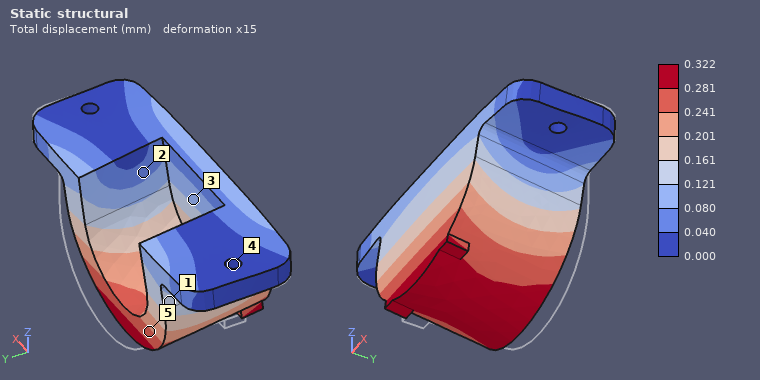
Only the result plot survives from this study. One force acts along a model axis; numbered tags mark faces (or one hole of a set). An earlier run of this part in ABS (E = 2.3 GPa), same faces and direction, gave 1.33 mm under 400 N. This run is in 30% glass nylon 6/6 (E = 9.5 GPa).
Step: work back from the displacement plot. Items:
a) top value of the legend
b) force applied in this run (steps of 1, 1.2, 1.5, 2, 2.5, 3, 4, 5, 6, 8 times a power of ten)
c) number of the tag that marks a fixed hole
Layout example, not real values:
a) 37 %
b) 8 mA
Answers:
a) 0.322 mm
b) 400 N
c) 4
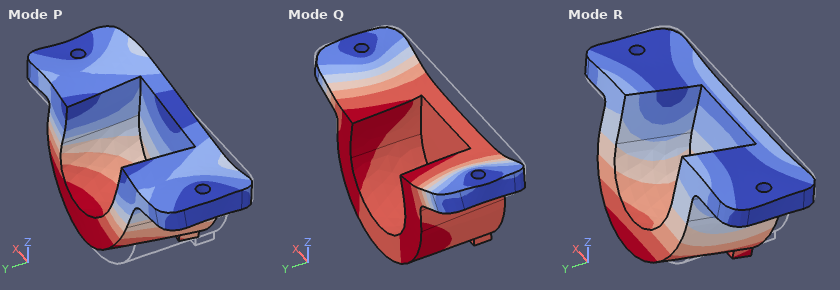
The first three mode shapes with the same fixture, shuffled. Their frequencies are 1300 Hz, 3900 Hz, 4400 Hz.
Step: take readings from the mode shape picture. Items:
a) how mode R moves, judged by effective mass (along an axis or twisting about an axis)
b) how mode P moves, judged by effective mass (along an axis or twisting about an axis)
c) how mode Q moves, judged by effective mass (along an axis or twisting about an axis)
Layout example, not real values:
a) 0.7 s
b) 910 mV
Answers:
a) along Y
b) along X
c) along Z
